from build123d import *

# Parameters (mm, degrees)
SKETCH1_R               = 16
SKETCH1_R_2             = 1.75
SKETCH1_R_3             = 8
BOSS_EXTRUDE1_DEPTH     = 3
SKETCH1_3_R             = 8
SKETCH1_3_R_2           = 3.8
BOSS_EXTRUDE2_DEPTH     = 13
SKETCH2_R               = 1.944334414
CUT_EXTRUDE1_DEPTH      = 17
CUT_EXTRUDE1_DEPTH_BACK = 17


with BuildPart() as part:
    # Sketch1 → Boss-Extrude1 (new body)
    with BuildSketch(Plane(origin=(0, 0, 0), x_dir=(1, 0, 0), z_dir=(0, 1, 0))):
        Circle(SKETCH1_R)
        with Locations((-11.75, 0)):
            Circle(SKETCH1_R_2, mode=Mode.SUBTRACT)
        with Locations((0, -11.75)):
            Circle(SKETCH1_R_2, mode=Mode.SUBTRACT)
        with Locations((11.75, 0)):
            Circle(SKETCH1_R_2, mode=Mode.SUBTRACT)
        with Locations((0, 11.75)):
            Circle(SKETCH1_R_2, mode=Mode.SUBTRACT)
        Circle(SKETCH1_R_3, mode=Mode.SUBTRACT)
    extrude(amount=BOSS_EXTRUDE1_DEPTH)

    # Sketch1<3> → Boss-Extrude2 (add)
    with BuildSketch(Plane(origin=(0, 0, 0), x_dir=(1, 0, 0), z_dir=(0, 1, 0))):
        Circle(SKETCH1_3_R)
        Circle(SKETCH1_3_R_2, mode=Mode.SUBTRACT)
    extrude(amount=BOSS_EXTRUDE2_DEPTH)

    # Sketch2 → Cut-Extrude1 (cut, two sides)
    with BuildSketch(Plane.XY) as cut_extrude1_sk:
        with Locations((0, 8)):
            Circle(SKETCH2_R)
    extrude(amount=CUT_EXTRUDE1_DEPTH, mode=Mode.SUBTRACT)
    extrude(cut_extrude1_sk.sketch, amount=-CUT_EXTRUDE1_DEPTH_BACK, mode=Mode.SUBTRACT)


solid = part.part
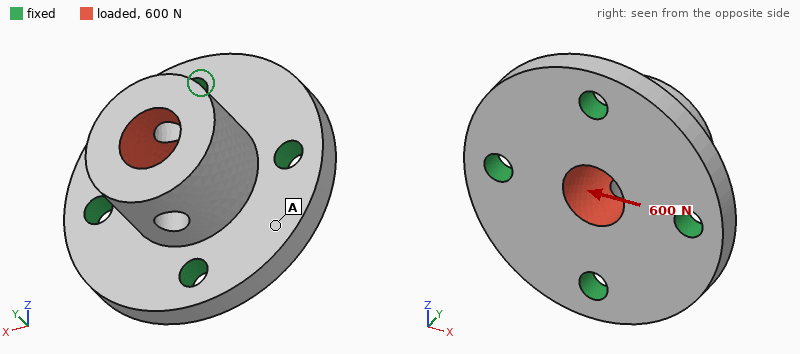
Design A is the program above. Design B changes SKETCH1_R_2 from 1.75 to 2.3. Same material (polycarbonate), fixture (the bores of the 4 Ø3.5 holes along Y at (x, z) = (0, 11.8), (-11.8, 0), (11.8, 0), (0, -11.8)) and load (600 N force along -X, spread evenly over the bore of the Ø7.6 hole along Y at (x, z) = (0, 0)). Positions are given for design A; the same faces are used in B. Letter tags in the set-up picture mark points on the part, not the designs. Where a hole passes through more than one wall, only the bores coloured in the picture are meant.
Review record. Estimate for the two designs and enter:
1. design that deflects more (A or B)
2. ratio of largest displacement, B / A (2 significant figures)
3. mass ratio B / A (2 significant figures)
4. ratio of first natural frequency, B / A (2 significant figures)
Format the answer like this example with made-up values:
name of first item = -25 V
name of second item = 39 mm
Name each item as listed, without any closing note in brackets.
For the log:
design that deflects more = A
ratio of largest displacement, B / A = 0.88
mass ratio B / A = 0.98
ratio of first natural frequency, B / A = 1.1
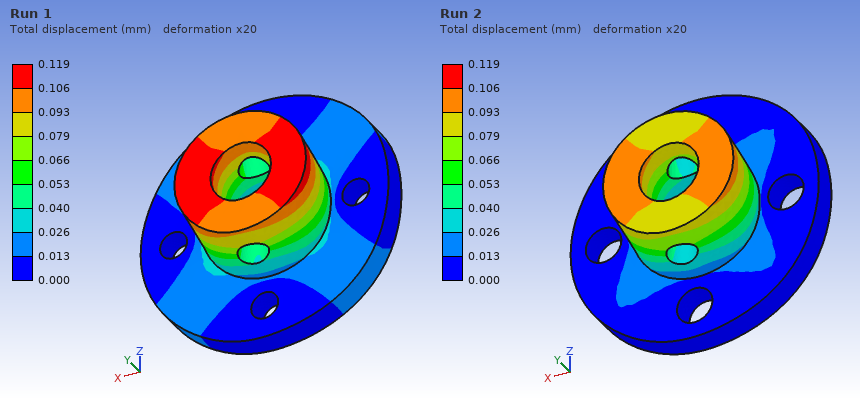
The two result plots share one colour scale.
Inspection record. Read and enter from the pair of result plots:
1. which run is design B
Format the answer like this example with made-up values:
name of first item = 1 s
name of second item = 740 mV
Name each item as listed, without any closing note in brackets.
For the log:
which run is design B = Run 2
